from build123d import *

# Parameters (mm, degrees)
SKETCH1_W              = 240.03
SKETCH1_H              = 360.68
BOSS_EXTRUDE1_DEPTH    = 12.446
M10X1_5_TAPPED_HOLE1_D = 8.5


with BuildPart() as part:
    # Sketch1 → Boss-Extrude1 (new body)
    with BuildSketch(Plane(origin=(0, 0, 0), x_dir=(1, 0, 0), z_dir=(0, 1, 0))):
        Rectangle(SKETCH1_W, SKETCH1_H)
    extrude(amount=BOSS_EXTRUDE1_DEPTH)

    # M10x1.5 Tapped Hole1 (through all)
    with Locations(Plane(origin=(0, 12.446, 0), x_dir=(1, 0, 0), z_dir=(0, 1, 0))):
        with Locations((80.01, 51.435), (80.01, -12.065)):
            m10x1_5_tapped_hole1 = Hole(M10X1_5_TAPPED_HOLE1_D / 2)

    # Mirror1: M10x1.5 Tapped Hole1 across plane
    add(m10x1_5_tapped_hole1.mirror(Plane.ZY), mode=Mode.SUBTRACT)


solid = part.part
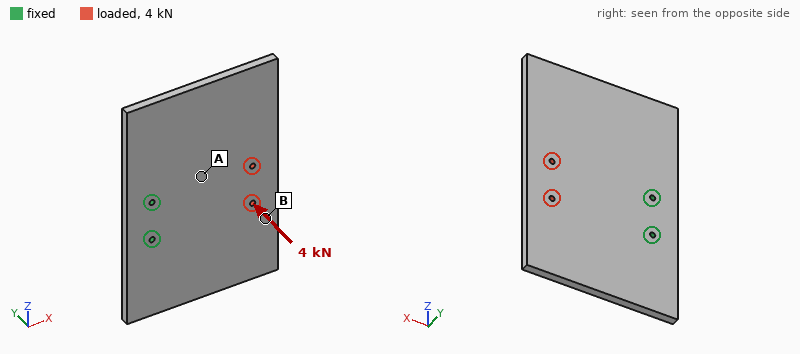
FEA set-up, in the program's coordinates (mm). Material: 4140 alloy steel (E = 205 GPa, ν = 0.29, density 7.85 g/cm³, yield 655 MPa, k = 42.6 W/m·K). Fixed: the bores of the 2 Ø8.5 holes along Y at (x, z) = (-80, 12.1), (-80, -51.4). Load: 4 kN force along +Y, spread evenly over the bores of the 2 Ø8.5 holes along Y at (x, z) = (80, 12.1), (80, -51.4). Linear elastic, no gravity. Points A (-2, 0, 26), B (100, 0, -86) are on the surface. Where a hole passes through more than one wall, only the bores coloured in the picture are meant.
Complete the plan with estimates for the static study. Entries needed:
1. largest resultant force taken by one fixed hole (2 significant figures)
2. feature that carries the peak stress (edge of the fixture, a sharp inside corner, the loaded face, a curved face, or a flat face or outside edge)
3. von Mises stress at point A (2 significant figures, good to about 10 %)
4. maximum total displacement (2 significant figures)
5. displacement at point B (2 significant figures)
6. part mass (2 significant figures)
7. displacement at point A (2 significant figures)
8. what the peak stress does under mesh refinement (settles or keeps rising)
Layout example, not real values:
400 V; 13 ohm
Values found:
2.0 kN; edge of the fixture; 40 MPa; 1.1 mm; 0.98 mm; 8.4 kg; 0.31 mm; keeps rising
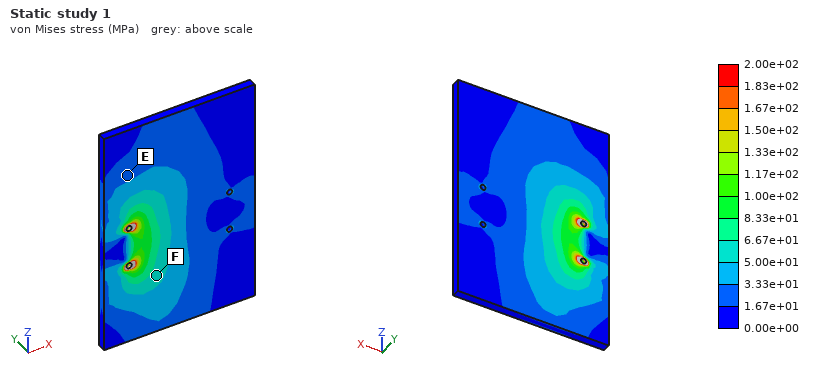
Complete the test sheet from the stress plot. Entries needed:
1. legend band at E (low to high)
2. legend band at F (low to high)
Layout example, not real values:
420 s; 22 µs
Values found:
1.67e+01 to 3.33e+01 MPa; 5.00e+01 to 6.67e+01 MPa
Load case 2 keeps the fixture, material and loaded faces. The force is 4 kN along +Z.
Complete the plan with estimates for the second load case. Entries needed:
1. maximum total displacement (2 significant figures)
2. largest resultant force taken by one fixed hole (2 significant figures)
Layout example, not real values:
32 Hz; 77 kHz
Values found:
36 µm; 9.6 kN
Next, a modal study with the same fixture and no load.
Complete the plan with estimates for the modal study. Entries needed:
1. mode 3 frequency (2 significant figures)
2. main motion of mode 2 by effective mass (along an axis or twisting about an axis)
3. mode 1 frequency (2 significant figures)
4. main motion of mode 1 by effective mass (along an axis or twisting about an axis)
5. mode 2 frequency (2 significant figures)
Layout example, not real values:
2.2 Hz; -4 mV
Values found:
440 Hz; twisting about X; 180 Hz; along Y; 240 Hz
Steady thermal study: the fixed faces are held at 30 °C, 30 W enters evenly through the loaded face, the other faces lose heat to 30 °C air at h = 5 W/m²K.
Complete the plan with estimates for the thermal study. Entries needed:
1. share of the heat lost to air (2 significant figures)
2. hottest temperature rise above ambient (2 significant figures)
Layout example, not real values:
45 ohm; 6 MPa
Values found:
46 %; 38 K
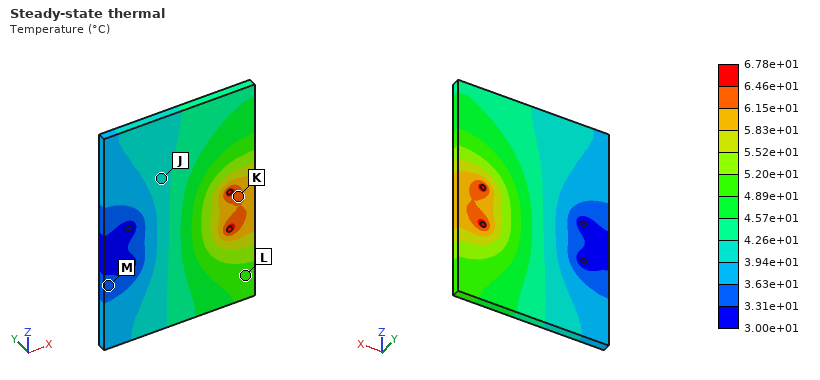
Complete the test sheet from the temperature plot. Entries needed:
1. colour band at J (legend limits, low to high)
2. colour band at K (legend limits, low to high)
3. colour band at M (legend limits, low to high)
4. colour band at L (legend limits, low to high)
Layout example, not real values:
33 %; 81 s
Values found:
3.94e+01 to 4.26e+01 °C; 6.15e+01 to 6.46e+01 °C; 3.31e+01 to 3.63e+01 °C; 4.89e+01 to 5.20e+01 °C
